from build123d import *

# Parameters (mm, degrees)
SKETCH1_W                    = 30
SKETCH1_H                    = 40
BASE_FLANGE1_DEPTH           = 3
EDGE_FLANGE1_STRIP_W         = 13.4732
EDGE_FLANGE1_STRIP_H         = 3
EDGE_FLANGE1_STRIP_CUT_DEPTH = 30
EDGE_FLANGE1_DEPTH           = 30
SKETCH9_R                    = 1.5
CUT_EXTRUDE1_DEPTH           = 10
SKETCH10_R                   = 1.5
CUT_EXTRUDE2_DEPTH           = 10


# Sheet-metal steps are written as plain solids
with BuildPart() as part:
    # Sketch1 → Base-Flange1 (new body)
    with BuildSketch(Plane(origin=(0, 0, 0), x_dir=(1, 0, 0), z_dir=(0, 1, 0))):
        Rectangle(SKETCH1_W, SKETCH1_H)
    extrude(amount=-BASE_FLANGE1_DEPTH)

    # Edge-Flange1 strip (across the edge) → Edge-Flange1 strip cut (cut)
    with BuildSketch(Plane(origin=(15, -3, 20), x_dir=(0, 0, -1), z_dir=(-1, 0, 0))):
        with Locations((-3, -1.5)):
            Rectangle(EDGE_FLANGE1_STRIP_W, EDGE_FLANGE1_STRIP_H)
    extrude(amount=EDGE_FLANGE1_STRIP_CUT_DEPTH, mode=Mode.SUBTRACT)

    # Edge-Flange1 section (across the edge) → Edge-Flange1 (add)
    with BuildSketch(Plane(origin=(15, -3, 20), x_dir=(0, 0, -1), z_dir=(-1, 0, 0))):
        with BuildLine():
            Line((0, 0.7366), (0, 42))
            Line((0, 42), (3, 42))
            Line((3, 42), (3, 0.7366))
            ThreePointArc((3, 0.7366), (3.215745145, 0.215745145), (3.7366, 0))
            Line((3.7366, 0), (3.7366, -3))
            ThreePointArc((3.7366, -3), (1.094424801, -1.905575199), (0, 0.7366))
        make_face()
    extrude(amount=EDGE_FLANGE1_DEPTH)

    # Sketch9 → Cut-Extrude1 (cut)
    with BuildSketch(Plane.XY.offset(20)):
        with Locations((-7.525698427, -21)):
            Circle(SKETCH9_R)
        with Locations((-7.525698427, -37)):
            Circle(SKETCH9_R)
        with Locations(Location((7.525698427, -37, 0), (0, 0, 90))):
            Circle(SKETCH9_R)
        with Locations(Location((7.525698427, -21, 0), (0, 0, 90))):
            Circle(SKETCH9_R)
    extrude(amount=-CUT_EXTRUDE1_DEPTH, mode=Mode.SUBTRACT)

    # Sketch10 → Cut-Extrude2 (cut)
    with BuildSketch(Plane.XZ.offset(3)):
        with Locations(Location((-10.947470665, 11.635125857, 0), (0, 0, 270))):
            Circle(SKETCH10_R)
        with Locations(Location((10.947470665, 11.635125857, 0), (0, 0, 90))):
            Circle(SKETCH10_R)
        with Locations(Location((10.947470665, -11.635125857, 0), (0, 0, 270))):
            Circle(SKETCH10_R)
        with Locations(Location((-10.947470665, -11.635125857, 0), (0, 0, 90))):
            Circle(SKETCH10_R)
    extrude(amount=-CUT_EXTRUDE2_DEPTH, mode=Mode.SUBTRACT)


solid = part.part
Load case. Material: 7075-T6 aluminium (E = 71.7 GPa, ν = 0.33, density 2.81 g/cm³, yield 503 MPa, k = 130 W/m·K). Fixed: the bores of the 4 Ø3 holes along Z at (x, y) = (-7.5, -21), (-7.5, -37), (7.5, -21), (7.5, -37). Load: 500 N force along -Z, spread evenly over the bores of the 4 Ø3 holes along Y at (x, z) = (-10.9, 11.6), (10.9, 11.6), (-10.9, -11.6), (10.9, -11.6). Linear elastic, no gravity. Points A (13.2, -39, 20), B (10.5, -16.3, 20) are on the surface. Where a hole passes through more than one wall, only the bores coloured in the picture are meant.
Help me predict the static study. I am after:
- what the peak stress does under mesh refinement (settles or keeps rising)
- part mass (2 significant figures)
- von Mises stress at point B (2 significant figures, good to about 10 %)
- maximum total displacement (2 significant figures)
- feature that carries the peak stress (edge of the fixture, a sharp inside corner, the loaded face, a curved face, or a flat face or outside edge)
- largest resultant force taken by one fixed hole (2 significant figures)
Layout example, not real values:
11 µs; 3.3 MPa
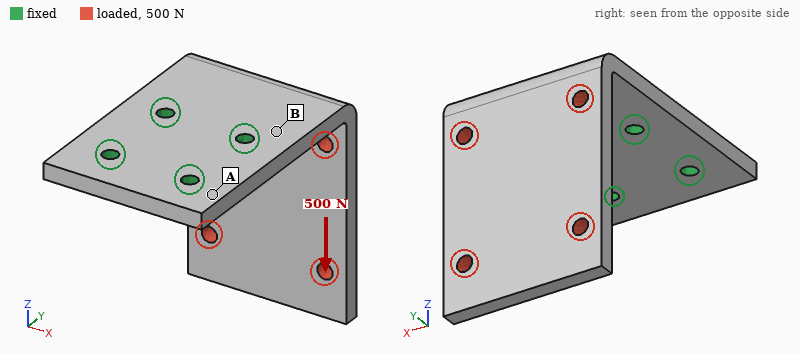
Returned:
keeps rising; 20 g; 150 MPa; 0.76 mm; edge of the fixture; 320 N
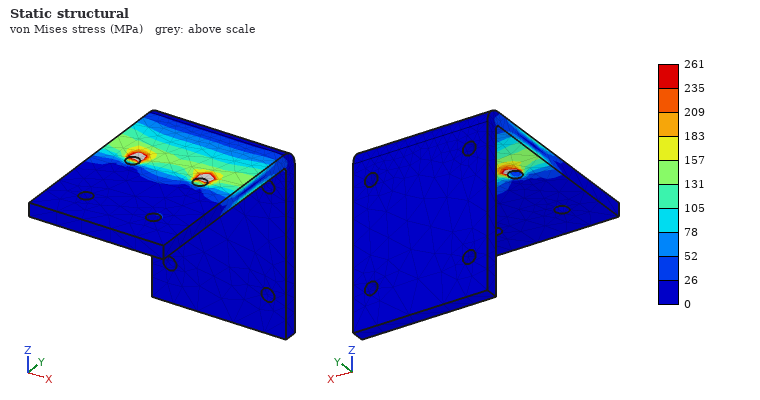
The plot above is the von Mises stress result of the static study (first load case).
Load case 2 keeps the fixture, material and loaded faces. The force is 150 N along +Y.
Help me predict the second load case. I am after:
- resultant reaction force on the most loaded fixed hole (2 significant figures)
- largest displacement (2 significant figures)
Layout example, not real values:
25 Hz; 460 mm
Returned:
69 N; 0.61 mm
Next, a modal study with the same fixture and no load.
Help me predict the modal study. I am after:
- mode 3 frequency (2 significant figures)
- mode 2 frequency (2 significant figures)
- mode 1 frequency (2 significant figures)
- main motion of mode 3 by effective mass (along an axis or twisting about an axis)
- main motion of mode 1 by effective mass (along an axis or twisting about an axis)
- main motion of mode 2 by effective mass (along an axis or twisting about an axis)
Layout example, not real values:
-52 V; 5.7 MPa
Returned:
3200 Hz; 1700 Hz; 940 Hz; along Z; along Y; along X
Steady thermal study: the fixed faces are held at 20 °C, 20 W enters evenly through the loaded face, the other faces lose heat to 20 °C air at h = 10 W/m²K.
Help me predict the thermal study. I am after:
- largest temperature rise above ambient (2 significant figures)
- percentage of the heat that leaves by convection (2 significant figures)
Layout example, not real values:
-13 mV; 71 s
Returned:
64 K; 7.6 %
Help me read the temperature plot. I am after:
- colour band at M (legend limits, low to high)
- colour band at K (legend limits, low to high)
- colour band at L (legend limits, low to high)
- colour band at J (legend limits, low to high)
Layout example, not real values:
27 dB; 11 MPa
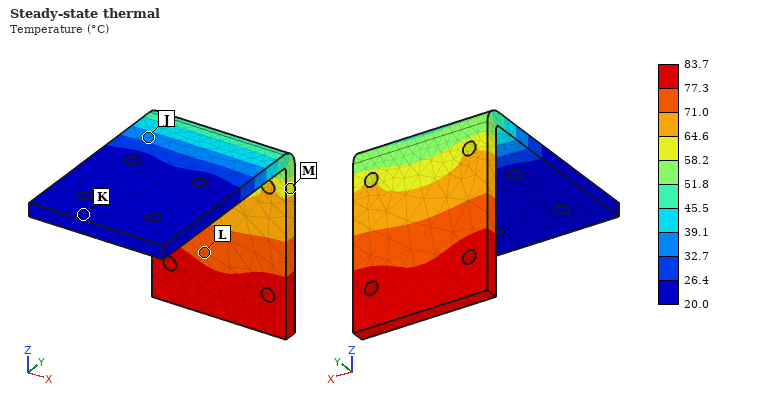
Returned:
58.2 to 64.6 °C; 20.0 to 26.4 °C; 71.0 to 77.3 °C; 32.7 to 39.1 °C
